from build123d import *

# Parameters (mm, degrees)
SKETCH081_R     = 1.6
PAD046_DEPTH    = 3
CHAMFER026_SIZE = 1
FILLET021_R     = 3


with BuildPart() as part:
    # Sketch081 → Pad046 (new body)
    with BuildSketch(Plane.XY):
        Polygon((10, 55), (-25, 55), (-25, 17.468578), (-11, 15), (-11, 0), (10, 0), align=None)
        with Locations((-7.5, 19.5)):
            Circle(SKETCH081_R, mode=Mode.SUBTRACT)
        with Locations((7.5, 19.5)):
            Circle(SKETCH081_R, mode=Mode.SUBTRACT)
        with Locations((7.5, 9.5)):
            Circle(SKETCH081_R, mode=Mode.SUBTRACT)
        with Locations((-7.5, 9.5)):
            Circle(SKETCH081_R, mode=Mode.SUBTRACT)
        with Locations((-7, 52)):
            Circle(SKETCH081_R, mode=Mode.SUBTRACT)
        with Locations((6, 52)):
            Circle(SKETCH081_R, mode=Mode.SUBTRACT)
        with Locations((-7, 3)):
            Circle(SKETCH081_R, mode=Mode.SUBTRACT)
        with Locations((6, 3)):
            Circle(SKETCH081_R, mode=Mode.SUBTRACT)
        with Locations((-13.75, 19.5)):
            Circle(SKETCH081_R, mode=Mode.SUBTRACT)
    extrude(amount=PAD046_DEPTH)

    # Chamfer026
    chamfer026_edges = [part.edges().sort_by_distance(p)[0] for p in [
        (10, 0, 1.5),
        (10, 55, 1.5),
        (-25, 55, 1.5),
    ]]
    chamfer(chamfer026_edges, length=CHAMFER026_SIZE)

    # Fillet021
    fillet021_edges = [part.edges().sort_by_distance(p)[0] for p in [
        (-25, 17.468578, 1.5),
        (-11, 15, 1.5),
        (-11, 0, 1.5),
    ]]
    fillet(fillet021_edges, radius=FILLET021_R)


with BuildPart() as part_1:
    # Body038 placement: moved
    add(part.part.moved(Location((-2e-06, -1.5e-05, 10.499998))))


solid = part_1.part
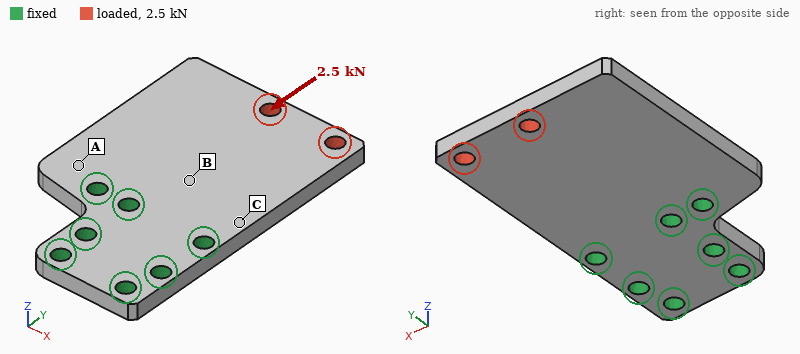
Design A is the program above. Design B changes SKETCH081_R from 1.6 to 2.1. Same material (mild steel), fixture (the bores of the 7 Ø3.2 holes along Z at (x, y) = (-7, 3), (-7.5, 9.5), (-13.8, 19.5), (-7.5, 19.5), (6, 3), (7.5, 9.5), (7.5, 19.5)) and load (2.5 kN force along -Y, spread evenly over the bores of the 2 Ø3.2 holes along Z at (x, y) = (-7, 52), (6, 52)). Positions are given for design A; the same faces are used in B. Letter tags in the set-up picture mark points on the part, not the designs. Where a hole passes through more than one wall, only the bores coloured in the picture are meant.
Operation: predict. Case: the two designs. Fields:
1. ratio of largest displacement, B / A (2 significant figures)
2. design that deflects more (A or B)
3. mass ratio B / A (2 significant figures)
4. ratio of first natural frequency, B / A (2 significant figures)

1.1
B
0.97
1.1
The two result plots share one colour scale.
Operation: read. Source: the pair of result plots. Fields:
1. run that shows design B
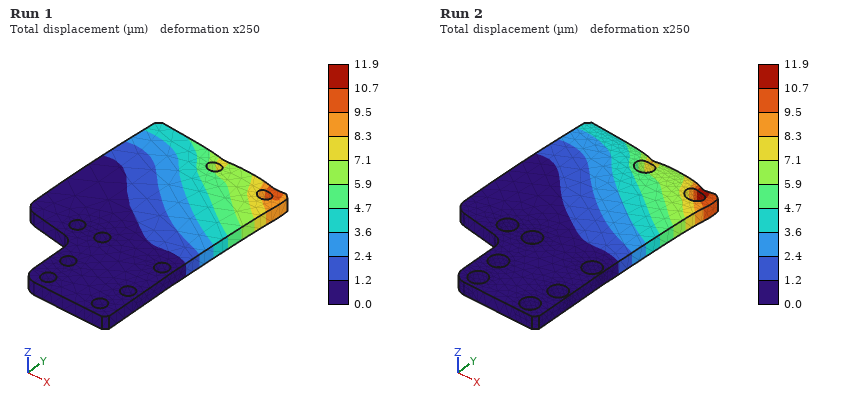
Run 2
